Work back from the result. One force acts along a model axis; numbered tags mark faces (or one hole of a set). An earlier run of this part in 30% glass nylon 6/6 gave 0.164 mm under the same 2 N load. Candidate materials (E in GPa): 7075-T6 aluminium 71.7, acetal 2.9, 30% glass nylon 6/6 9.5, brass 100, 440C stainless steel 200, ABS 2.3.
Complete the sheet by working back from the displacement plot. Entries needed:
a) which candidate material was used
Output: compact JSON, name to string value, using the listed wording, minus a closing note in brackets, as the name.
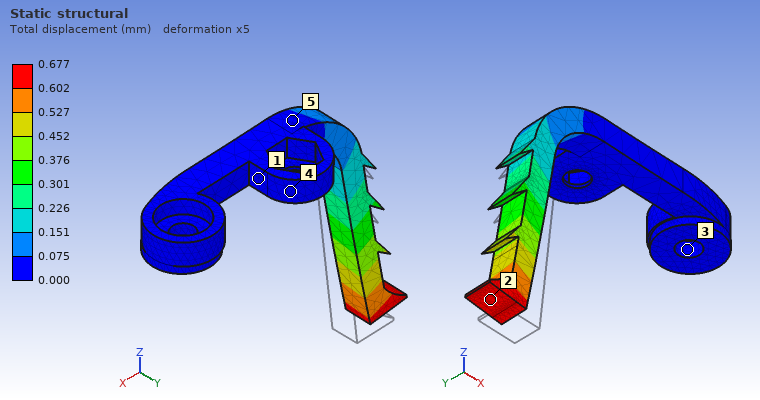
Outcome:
{"which candidate material was used": "ABS"}
